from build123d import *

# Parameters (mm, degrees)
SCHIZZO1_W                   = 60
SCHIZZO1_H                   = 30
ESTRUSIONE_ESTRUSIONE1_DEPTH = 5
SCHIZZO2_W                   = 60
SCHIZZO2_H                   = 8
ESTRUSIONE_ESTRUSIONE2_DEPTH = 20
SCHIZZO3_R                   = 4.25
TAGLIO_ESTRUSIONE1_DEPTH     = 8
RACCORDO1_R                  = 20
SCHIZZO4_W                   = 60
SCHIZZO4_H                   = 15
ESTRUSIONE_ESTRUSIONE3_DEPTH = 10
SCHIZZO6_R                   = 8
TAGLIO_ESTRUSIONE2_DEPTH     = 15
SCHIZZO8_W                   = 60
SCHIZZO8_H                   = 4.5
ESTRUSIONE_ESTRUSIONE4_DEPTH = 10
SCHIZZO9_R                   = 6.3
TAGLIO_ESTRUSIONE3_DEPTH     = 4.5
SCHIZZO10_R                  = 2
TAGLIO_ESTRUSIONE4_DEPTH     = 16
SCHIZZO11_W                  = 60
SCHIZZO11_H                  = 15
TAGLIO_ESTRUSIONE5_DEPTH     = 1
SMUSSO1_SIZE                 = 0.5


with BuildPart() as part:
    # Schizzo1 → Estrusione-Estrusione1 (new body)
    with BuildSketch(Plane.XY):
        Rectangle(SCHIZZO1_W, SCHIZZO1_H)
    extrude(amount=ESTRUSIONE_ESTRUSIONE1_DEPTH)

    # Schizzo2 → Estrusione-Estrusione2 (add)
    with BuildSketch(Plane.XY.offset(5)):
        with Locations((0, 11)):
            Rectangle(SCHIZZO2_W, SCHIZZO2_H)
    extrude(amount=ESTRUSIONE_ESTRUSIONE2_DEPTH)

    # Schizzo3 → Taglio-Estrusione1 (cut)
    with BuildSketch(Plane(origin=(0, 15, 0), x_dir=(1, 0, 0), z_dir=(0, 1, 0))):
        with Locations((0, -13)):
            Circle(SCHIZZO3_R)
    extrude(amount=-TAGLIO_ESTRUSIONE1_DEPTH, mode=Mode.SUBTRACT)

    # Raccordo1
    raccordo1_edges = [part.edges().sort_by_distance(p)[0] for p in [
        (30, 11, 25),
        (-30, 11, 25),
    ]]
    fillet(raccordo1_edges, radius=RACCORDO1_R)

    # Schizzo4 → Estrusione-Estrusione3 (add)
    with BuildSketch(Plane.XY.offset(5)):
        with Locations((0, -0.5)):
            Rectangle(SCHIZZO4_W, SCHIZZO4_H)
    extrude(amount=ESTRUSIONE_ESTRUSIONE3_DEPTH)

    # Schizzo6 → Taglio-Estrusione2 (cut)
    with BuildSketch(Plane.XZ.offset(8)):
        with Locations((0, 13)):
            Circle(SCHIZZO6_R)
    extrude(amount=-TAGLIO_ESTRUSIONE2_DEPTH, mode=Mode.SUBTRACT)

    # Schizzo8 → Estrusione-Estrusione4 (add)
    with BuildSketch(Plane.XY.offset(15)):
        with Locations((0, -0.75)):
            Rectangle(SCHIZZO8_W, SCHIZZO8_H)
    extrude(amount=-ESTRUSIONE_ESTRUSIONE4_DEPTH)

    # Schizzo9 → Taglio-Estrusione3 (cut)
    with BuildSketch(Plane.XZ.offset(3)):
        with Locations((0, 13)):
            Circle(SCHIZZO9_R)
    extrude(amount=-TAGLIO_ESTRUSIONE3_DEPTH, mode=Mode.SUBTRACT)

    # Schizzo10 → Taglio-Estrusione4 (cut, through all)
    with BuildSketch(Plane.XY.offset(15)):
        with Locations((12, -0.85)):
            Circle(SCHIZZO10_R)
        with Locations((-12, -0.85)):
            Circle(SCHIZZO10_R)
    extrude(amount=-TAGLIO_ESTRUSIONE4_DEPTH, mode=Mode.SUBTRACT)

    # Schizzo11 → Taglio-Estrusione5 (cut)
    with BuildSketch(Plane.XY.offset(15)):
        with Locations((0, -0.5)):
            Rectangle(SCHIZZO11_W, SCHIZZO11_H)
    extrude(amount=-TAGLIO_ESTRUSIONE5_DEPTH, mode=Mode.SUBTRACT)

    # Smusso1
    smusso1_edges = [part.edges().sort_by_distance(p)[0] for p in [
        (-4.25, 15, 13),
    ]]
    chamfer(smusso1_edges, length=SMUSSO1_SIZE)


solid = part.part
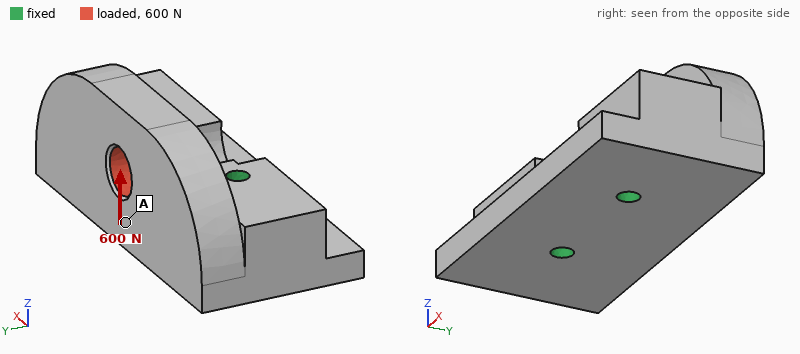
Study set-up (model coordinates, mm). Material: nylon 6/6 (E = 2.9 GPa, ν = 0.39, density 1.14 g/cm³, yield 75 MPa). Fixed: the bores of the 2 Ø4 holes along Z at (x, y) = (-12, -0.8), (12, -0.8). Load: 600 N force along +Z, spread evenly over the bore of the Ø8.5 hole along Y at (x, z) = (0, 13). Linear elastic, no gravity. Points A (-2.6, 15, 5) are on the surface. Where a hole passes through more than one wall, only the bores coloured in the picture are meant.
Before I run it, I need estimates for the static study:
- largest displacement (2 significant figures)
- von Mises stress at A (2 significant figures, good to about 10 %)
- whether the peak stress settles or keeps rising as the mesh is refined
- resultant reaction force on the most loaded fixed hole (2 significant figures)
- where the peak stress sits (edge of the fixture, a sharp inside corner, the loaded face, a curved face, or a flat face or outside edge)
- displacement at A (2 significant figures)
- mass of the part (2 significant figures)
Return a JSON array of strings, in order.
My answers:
["78 µm", "2.8 MPa", "keeps rising", "300 N", "edge of the fixture", "57 µm", "26 g"]
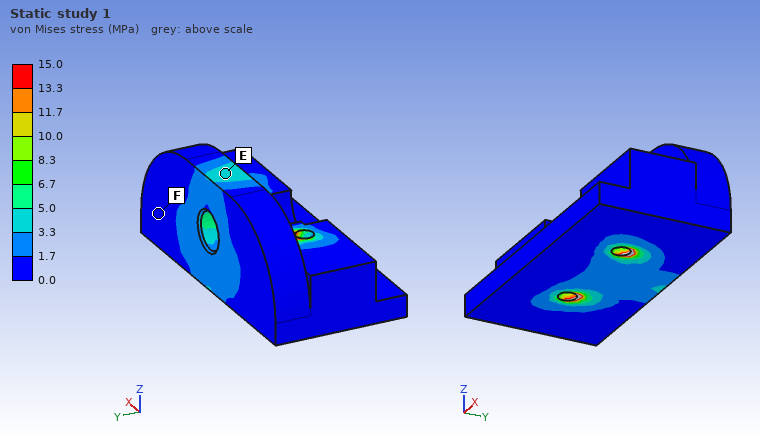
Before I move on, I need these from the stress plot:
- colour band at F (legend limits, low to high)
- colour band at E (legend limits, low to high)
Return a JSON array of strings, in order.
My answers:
["0.0 to 1.7 MPa", "3.3 to 5.0 MPa"]
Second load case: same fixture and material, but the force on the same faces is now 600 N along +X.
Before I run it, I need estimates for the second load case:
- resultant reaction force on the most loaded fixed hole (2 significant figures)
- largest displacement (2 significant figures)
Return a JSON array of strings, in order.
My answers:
["380 N", "47 µm"]
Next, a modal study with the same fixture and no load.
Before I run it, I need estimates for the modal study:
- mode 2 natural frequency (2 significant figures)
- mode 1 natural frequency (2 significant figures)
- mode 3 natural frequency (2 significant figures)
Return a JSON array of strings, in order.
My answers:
["4800 Hz", "4600 Hz", "5500 Hz"]
